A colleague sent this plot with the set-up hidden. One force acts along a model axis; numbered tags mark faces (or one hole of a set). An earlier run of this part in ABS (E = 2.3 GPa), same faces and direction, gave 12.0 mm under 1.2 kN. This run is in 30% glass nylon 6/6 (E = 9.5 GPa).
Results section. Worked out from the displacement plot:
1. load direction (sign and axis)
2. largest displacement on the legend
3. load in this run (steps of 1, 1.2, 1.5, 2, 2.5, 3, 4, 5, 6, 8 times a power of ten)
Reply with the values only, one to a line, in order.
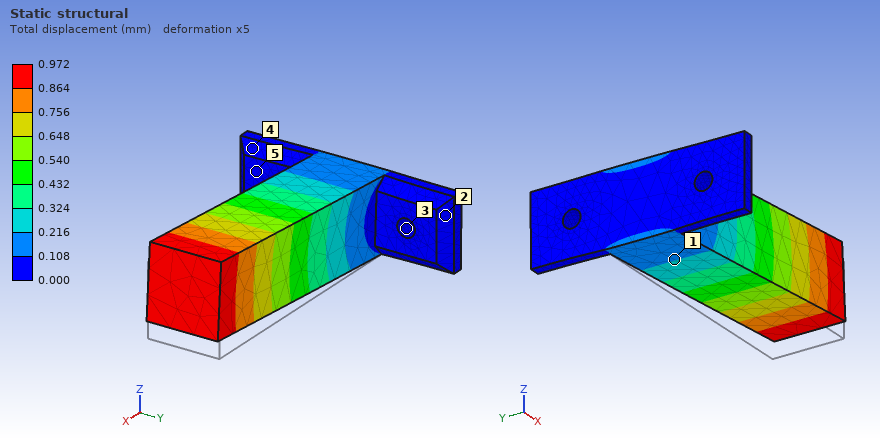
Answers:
+Z
0.972 mm
400 N
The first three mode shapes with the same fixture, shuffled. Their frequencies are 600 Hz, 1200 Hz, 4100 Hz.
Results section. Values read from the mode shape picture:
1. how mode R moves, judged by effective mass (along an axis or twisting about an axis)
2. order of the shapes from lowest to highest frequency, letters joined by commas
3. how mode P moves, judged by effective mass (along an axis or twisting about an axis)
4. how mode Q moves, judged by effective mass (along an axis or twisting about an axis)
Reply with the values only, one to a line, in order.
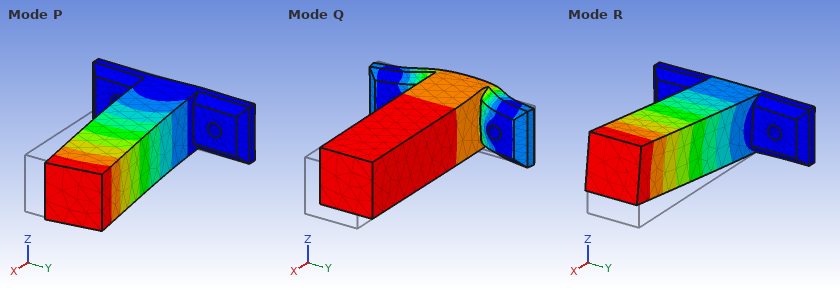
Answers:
along Z
R, P, Q
along Y
along X
